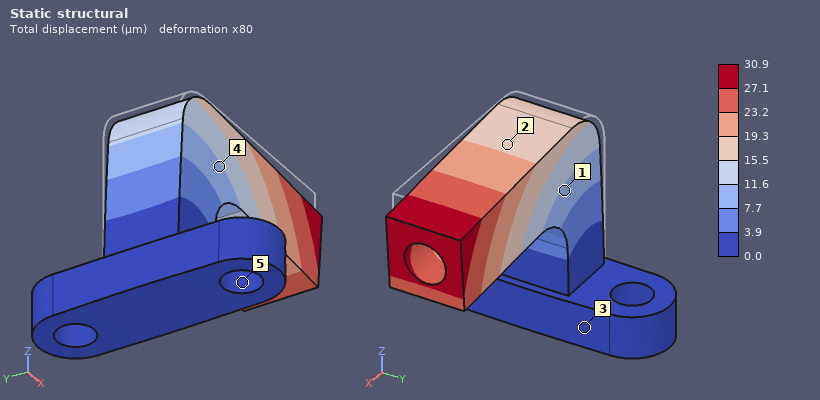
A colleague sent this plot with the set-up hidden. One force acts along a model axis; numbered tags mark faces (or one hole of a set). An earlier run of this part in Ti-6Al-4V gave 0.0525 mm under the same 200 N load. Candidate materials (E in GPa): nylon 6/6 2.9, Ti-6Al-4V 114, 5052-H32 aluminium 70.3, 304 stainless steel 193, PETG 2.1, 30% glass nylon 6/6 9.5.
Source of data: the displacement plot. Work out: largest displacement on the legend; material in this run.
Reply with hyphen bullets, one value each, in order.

- 30.9 µm
- 304 stainless steel
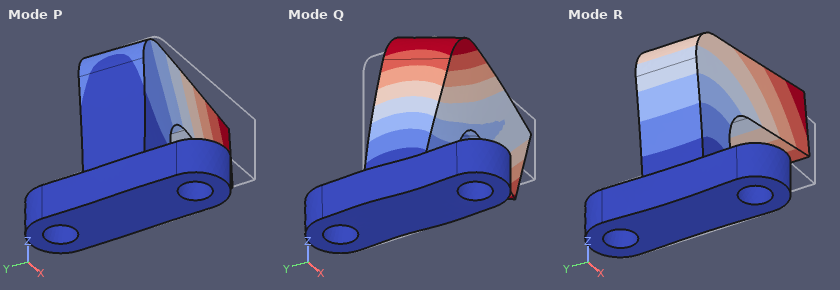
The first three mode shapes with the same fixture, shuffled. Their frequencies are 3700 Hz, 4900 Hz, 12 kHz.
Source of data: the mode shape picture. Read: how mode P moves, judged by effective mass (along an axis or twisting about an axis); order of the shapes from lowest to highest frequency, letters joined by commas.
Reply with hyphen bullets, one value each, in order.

- along Y
- R, P, Q
